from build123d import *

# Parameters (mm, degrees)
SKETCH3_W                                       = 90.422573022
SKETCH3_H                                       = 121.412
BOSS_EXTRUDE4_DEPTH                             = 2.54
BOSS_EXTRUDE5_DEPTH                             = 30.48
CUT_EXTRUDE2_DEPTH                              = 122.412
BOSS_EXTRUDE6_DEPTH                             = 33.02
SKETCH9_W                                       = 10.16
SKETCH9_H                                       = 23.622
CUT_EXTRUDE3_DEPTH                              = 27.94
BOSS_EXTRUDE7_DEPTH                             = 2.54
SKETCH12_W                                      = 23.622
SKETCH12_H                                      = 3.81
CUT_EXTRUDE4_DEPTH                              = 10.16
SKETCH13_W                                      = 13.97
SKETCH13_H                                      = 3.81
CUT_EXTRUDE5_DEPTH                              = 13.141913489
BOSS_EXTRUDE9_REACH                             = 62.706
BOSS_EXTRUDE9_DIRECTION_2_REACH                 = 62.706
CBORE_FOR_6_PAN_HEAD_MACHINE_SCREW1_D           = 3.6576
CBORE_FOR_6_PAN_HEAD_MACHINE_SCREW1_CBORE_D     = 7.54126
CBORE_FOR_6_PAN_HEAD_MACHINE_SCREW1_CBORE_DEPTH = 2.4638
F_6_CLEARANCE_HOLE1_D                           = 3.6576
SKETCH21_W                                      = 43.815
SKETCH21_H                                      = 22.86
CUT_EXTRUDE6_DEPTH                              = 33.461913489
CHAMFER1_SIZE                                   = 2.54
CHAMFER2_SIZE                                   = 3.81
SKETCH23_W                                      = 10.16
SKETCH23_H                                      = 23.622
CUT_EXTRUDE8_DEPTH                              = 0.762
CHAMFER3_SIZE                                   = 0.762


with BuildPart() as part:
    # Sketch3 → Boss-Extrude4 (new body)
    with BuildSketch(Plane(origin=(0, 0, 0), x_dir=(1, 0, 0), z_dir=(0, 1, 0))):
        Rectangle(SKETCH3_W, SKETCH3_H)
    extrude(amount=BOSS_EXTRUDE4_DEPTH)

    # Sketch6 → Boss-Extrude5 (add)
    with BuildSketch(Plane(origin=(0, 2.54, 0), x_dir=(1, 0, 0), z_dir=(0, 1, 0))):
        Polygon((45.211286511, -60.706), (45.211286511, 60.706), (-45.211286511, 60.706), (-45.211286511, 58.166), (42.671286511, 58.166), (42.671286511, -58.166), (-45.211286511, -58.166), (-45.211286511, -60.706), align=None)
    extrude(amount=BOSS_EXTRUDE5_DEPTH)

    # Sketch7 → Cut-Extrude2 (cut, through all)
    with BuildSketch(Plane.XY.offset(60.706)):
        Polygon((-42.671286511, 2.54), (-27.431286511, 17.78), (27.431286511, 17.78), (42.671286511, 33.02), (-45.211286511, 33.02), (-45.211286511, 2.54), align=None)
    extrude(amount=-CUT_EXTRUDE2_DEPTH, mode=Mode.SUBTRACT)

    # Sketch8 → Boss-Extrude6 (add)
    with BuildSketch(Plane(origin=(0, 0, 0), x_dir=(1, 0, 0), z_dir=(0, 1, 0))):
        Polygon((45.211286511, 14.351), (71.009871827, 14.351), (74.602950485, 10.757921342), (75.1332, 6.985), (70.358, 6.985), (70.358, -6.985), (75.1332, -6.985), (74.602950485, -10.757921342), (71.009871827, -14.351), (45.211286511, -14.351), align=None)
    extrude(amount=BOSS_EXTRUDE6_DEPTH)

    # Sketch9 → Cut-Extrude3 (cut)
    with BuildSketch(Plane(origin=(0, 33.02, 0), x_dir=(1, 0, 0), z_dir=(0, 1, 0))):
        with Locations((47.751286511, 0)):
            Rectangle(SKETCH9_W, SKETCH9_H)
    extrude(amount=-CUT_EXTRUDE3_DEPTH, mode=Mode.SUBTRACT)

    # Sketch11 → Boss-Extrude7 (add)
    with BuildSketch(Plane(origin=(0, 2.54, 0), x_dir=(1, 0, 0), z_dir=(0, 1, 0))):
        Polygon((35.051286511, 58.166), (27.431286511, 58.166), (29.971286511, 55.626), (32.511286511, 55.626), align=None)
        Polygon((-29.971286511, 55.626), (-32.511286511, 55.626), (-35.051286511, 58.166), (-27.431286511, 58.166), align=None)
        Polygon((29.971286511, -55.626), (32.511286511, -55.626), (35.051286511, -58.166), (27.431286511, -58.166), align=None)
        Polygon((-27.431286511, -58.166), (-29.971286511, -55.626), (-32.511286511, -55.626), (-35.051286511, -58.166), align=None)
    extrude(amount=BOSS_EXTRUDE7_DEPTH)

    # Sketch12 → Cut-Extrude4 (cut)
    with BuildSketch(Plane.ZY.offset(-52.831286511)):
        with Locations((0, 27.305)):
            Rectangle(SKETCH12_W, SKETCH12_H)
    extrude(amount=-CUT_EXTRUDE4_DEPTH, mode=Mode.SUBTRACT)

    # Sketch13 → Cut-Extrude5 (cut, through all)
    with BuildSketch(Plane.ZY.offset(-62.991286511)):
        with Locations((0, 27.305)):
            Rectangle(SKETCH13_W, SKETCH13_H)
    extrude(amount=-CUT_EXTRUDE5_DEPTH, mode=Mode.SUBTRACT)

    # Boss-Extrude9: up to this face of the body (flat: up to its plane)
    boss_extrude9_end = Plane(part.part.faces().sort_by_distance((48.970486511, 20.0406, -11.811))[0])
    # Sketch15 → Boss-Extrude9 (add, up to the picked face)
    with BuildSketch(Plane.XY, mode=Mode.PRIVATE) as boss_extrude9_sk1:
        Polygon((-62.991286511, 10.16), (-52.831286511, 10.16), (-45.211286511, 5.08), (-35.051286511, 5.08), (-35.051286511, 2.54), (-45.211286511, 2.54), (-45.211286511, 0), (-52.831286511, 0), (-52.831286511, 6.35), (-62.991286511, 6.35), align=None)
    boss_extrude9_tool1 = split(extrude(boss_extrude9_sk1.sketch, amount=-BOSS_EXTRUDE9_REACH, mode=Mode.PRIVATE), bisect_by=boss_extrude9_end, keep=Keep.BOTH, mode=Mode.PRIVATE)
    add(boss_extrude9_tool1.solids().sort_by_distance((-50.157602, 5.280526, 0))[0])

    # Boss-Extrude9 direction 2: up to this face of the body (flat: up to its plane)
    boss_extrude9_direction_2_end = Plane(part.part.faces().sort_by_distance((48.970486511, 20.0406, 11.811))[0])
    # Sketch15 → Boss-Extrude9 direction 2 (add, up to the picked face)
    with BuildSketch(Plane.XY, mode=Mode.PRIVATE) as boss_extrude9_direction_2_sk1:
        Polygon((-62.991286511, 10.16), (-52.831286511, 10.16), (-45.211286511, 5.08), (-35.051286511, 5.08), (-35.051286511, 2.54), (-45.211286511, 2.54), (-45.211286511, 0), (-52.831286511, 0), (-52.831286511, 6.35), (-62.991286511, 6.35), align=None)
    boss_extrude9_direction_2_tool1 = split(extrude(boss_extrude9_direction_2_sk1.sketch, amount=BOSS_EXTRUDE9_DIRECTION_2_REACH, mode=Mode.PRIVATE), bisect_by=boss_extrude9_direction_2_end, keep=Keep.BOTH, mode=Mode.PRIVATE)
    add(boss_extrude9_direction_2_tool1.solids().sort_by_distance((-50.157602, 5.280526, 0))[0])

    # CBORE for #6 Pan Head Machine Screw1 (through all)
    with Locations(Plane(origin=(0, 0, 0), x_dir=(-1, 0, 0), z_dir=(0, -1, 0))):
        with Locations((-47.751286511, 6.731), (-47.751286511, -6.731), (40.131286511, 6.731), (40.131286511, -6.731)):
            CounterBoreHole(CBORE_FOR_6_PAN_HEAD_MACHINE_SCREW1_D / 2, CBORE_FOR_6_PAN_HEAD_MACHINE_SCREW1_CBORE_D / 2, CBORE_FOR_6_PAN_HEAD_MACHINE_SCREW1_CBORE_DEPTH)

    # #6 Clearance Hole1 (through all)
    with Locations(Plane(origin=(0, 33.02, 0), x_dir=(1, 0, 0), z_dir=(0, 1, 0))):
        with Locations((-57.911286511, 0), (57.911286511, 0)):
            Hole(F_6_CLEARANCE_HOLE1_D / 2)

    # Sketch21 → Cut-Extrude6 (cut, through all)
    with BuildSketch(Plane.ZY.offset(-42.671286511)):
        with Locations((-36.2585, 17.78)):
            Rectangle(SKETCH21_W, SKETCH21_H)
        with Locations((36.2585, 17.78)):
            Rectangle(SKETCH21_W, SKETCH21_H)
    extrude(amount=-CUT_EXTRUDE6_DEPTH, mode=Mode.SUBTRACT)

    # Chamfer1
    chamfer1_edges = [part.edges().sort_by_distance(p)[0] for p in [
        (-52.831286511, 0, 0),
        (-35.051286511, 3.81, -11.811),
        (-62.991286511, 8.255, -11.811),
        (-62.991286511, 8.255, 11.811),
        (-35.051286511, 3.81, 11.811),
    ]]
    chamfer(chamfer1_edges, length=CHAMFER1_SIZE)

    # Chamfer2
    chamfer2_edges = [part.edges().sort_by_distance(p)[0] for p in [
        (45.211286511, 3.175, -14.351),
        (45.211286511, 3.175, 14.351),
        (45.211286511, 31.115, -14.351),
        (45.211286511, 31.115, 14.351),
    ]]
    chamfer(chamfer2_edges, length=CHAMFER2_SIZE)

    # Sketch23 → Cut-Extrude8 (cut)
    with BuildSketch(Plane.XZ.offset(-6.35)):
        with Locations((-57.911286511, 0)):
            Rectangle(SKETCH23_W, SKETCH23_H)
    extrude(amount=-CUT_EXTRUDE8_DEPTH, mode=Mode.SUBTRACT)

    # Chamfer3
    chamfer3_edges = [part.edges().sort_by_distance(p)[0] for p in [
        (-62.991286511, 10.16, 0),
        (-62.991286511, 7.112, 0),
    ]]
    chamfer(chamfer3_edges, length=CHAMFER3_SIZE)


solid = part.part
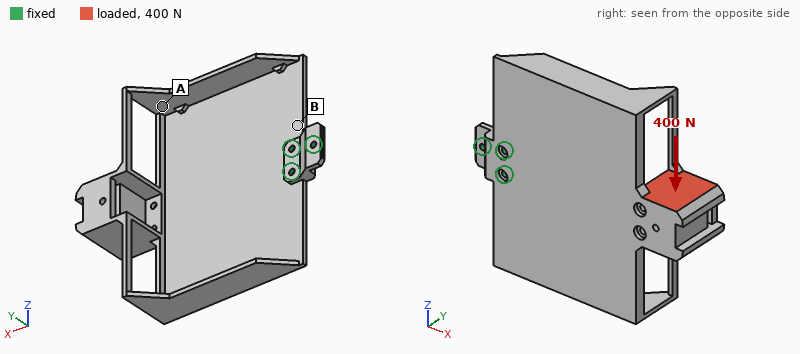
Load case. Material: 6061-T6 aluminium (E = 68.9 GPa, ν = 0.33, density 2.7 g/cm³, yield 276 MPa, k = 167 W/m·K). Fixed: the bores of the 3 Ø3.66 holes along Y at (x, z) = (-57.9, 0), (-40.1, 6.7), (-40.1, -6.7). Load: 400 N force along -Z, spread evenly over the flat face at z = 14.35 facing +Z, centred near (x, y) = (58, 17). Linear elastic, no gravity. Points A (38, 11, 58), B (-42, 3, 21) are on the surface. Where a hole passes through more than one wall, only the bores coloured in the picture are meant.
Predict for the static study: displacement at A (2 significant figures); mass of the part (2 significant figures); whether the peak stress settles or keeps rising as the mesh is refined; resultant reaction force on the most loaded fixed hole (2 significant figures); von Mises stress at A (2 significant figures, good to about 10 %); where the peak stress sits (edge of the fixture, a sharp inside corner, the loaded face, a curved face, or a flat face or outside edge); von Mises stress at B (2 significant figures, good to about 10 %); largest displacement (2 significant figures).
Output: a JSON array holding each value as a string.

["1.7 mm", "160 g", "keeps rising", "1.6 kN", "19 MPa", "edge of the fixture", "51 MPa", "2.1 mm"]
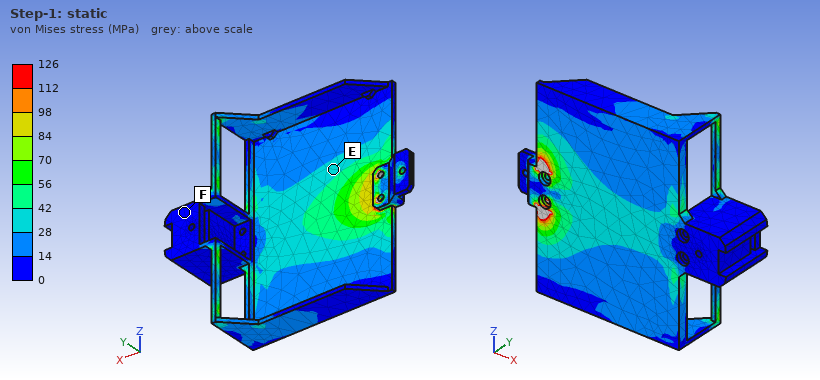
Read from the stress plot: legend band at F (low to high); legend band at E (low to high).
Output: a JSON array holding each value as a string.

["0 to 14 MPa", "28 to 42 MPa"]
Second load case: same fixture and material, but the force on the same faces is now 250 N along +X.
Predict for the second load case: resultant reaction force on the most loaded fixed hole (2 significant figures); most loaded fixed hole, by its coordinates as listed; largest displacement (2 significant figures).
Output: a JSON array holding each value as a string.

["350 N", "(-40.1, 6.7)", "2.1 mm"]
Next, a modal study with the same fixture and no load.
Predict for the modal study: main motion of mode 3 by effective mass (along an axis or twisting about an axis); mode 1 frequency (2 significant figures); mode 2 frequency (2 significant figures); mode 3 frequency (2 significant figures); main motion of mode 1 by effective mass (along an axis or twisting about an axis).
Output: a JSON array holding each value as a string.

["along Y", "100 Hz", "210 Hz", "550 Hz", "along Y"]
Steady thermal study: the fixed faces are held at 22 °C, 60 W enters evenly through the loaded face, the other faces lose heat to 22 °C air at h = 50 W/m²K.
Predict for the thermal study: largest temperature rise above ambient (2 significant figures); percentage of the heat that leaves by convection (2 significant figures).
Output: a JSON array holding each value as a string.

["79 K", "84 %"]
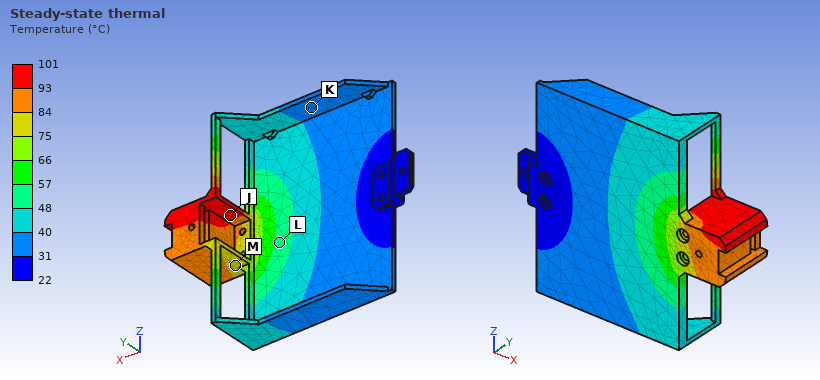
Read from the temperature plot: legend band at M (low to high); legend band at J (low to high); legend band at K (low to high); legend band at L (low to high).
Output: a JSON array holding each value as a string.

["75 to 84 °C", "93 to 101 °C", "31 to 40 °C", "48 to 57 °C"]
